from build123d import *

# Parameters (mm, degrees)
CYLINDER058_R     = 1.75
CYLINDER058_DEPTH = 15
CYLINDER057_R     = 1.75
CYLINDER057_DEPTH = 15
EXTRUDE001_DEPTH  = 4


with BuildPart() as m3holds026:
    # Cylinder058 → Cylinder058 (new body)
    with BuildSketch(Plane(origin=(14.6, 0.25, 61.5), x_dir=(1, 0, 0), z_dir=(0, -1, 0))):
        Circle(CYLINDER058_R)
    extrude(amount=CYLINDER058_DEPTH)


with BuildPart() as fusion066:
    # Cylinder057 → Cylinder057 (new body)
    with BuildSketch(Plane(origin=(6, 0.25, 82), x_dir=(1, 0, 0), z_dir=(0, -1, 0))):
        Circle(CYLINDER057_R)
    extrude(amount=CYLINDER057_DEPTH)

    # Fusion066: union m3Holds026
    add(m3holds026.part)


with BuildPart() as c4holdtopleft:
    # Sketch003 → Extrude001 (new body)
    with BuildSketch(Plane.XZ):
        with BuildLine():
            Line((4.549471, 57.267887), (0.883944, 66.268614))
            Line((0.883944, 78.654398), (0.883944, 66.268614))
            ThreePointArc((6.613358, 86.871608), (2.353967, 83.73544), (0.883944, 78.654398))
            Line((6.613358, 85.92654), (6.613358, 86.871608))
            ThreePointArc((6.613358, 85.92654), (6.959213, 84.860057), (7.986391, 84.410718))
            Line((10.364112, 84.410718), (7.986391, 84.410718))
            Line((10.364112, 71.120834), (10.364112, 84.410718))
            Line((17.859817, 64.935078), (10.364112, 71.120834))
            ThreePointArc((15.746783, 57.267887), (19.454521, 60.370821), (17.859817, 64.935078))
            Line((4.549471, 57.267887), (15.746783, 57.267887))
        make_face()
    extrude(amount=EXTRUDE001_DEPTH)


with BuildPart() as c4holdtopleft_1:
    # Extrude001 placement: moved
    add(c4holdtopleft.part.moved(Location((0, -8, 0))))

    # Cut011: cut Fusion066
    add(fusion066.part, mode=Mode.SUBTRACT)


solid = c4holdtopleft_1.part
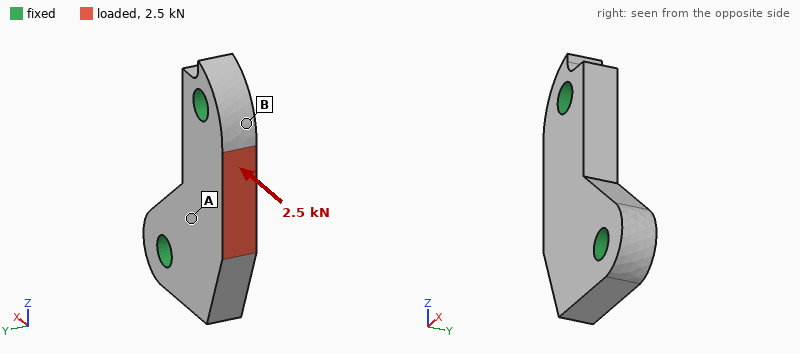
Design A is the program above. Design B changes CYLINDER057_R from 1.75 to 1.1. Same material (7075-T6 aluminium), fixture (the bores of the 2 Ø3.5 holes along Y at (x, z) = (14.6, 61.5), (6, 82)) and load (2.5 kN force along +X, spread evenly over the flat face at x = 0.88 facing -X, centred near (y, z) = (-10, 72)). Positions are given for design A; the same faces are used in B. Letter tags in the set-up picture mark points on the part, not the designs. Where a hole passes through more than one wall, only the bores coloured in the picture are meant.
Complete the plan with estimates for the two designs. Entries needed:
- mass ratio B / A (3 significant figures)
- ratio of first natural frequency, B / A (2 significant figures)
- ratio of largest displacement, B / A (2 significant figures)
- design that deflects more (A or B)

1.02
0.95
1.1
B
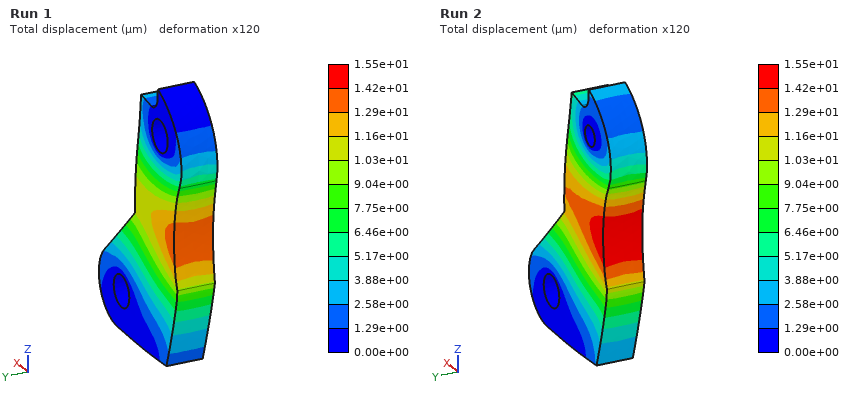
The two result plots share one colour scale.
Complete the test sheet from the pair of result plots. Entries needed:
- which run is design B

Run 2
